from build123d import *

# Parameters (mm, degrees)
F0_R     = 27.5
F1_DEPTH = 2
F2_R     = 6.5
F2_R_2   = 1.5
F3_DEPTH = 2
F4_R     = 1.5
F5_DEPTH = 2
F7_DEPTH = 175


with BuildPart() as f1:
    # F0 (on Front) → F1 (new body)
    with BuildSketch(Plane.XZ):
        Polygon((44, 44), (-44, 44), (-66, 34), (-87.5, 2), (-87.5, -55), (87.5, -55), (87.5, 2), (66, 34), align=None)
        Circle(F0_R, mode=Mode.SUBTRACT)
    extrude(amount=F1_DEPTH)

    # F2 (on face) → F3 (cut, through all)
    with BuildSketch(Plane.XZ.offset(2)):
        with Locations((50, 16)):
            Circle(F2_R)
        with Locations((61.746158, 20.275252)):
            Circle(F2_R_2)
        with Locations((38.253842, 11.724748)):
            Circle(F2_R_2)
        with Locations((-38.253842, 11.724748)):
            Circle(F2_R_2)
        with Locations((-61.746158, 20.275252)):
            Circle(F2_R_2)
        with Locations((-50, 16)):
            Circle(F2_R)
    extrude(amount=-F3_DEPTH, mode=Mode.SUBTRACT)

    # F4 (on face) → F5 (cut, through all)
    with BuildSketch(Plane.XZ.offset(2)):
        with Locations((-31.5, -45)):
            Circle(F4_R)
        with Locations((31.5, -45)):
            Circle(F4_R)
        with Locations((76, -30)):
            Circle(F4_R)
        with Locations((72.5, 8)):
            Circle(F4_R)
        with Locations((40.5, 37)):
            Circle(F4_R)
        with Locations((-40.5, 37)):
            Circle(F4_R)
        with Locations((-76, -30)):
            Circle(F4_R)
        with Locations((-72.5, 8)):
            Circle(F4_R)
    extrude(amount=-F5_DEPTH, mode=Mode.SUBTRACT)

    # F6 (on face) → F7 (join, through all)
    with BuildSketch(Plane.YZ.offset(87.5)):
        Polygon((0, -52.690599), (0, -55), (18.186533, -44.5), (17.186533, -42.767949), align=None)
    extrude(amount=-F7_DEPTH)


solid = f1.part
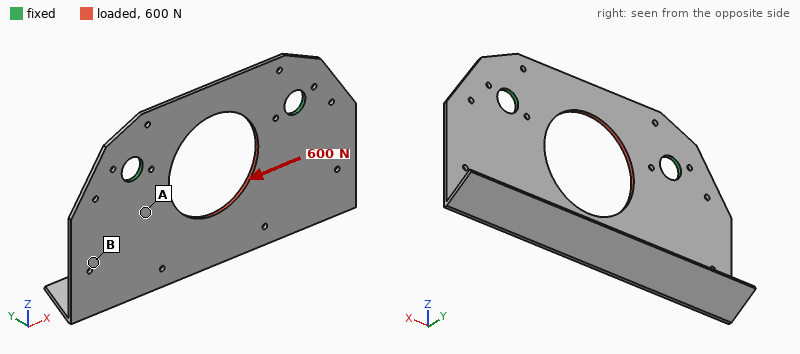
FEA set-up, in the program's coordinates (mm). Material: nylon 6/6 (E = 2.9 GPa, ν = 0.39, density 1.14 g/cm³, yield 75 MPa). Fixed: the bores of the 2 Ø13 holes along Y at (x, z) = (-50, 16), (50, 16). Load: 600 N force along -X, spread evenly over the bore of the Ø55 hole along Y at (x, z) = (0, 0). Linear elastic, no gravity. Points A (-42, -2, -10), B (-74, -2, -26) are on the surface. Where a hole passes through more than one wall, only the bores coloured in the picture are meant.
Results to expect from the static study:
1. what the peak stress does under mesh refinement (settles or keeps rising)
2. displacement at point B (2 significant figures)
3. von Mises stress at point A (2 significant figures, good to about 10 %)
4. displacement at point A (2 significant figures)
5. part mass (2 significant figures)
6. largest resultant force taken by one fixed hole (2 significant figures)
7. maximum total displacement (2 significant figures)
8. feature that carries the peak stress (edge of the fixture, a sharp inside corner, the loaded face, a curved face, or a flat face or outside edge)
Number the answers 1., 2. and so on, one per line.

1. keeps rising
2. 0.11 mm
3. 3.1 MPa
4. 0.079 mm
5. 38 g
6. 310 N
7. 0.16 mm
8. edge of the fixture
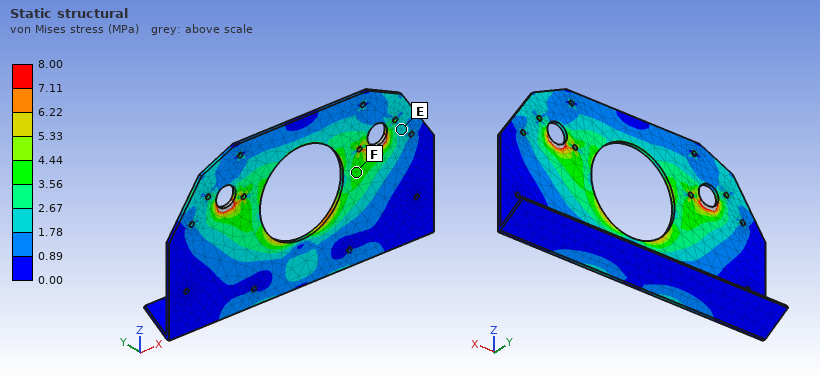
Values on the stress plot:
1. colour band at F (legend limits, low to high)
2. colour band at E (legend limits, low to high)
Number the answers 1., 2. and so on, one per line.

1. 3.56 to 4.44 MPa
2. 1.78 to 2.67 MPa
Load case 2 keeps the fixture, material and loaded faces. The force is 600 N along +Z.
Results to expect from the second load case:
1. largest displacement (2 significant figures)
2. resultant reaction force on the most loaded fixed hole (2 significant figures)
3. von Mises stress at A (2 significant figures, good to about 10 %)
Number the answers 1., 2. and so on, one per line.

1. 0.13 mm
2. 300 N
3. 3.2 MPa
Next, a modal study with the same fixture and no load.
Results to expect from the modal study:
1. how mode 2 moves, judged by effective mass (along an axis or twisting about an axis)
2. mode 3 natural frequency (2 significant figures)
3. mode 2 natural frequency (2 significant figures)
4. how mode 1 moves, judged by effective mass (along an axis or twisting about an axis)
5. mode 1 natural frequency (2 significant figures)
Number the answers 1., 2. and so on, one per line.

1. twisting about Z
2. 380 Hz
3. 100 Hz
4. along Y
5. 67 Hz
